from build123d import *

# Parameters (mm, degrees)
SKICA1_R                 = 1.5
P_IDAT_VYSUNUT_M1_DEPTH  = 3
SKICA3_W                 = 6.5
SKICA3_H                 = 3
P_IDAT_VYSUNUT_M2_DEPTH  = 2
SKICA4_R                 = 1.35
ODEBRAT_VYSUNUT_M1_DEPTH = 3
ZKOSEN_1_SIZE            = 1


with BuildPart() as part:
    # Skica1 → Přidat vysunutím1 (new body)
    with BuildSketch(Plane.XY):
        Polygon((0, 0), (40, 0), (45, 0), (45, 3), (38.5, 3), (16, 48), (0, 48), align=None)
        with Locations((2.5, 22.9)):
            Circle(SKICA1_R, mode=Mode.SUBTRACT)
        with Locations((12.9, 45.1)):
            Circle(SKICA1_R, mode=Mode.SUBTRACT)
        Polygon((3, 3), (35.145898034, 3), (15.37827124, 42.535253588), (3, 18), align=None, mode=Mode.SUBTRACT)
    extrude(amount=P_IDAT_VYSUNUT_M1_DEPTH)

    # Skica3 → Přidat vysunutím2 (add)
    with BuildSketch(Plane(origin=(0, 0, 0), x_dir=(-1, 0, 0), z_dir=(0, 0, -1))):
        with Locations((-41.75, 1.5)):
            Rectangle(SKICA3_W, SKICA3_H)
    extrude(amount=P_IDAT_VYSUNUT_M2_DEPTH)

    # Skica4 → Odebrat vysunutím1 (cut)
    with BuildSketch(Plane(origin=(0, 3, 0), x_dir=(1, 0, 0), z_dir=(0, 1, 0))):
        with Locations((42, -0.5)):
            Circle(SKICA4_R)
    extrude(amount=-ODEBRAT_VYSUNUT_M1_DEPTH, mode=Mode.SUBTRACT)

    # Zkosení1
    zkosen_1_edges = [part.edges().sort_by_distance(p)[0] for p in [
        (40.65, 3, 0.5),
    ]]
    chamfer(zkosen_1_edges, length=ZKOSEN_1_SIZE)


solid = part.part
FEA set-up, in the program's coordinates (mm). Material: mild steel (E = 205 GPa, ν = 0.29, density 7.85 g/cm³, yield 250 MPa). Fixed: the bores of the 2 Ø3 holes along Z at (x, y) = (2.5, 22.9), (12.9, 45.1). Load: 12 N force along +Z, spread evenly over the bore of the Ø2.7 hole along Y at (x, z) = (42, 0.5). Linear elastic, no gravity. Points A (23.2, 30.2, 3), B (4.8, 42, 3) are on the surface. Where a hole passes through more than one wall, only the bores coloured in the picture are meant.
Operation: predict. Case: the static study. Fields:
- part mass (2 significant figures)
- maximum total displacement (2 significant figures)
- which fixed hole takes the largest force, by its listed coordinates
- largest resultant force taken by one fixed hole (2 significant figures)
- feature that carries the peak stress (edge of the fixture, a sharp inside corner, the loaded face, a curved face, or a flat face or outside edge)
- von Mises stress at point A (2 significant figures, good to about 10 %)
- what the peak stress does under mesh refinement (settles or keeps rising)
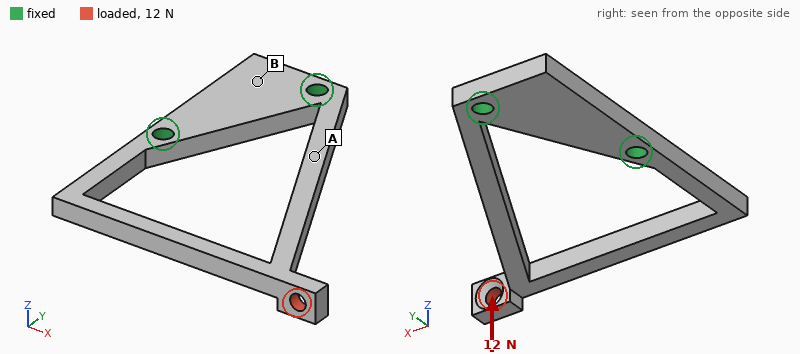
15 g
0.24 mm
(12.9, 45.1)
7.7 N
a sharp inside corner
50 MPa
keeps rising
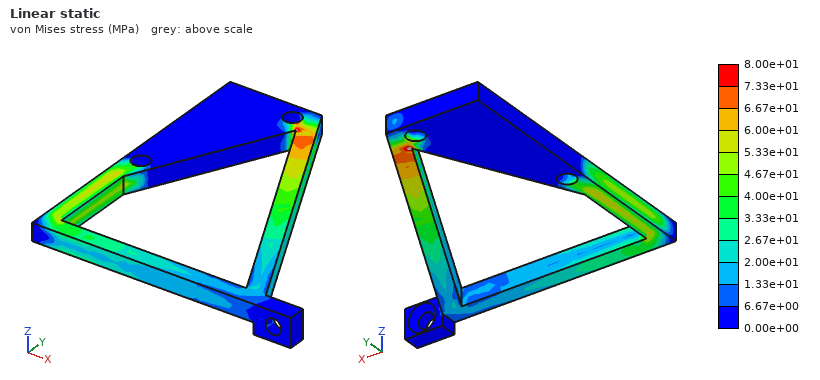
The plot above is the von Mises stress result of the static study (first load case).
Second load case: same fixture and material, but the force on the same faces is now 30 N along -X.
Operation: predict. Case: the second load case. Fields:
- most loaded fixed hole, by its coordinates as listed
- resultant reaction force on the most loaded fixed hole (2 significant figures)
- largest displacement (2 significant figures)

(2.5, 22.9)
34 N
38 µm
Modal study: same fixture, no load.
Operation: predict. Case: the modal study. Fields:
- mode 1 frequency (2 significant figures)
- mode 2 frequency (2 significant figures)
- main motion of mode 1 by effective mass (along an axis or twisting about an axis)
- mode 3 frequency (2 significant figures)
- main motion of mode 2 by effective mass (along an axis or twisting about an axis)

860 Hz
2200 Hz
along Z
3400 Hz
along X
